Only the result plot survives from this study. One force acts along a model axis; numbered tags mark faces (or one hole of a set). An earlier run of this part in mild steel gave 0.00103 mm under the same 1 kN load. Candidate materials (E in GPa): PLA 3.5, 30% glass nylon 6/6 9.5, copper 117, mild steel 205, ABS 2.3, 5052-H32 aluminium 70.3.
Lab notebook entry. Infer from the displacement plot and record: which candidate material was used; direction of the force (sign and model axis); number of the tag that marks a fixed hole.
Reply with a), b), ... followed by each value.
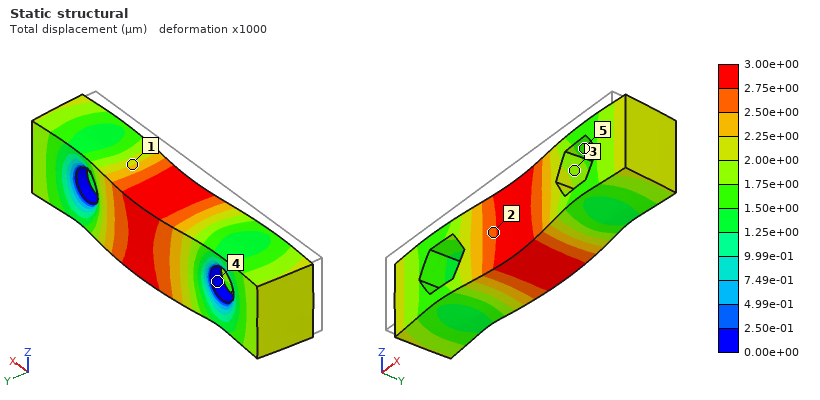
a) 5052-H32 aluminium
b) +Y
c) 4
